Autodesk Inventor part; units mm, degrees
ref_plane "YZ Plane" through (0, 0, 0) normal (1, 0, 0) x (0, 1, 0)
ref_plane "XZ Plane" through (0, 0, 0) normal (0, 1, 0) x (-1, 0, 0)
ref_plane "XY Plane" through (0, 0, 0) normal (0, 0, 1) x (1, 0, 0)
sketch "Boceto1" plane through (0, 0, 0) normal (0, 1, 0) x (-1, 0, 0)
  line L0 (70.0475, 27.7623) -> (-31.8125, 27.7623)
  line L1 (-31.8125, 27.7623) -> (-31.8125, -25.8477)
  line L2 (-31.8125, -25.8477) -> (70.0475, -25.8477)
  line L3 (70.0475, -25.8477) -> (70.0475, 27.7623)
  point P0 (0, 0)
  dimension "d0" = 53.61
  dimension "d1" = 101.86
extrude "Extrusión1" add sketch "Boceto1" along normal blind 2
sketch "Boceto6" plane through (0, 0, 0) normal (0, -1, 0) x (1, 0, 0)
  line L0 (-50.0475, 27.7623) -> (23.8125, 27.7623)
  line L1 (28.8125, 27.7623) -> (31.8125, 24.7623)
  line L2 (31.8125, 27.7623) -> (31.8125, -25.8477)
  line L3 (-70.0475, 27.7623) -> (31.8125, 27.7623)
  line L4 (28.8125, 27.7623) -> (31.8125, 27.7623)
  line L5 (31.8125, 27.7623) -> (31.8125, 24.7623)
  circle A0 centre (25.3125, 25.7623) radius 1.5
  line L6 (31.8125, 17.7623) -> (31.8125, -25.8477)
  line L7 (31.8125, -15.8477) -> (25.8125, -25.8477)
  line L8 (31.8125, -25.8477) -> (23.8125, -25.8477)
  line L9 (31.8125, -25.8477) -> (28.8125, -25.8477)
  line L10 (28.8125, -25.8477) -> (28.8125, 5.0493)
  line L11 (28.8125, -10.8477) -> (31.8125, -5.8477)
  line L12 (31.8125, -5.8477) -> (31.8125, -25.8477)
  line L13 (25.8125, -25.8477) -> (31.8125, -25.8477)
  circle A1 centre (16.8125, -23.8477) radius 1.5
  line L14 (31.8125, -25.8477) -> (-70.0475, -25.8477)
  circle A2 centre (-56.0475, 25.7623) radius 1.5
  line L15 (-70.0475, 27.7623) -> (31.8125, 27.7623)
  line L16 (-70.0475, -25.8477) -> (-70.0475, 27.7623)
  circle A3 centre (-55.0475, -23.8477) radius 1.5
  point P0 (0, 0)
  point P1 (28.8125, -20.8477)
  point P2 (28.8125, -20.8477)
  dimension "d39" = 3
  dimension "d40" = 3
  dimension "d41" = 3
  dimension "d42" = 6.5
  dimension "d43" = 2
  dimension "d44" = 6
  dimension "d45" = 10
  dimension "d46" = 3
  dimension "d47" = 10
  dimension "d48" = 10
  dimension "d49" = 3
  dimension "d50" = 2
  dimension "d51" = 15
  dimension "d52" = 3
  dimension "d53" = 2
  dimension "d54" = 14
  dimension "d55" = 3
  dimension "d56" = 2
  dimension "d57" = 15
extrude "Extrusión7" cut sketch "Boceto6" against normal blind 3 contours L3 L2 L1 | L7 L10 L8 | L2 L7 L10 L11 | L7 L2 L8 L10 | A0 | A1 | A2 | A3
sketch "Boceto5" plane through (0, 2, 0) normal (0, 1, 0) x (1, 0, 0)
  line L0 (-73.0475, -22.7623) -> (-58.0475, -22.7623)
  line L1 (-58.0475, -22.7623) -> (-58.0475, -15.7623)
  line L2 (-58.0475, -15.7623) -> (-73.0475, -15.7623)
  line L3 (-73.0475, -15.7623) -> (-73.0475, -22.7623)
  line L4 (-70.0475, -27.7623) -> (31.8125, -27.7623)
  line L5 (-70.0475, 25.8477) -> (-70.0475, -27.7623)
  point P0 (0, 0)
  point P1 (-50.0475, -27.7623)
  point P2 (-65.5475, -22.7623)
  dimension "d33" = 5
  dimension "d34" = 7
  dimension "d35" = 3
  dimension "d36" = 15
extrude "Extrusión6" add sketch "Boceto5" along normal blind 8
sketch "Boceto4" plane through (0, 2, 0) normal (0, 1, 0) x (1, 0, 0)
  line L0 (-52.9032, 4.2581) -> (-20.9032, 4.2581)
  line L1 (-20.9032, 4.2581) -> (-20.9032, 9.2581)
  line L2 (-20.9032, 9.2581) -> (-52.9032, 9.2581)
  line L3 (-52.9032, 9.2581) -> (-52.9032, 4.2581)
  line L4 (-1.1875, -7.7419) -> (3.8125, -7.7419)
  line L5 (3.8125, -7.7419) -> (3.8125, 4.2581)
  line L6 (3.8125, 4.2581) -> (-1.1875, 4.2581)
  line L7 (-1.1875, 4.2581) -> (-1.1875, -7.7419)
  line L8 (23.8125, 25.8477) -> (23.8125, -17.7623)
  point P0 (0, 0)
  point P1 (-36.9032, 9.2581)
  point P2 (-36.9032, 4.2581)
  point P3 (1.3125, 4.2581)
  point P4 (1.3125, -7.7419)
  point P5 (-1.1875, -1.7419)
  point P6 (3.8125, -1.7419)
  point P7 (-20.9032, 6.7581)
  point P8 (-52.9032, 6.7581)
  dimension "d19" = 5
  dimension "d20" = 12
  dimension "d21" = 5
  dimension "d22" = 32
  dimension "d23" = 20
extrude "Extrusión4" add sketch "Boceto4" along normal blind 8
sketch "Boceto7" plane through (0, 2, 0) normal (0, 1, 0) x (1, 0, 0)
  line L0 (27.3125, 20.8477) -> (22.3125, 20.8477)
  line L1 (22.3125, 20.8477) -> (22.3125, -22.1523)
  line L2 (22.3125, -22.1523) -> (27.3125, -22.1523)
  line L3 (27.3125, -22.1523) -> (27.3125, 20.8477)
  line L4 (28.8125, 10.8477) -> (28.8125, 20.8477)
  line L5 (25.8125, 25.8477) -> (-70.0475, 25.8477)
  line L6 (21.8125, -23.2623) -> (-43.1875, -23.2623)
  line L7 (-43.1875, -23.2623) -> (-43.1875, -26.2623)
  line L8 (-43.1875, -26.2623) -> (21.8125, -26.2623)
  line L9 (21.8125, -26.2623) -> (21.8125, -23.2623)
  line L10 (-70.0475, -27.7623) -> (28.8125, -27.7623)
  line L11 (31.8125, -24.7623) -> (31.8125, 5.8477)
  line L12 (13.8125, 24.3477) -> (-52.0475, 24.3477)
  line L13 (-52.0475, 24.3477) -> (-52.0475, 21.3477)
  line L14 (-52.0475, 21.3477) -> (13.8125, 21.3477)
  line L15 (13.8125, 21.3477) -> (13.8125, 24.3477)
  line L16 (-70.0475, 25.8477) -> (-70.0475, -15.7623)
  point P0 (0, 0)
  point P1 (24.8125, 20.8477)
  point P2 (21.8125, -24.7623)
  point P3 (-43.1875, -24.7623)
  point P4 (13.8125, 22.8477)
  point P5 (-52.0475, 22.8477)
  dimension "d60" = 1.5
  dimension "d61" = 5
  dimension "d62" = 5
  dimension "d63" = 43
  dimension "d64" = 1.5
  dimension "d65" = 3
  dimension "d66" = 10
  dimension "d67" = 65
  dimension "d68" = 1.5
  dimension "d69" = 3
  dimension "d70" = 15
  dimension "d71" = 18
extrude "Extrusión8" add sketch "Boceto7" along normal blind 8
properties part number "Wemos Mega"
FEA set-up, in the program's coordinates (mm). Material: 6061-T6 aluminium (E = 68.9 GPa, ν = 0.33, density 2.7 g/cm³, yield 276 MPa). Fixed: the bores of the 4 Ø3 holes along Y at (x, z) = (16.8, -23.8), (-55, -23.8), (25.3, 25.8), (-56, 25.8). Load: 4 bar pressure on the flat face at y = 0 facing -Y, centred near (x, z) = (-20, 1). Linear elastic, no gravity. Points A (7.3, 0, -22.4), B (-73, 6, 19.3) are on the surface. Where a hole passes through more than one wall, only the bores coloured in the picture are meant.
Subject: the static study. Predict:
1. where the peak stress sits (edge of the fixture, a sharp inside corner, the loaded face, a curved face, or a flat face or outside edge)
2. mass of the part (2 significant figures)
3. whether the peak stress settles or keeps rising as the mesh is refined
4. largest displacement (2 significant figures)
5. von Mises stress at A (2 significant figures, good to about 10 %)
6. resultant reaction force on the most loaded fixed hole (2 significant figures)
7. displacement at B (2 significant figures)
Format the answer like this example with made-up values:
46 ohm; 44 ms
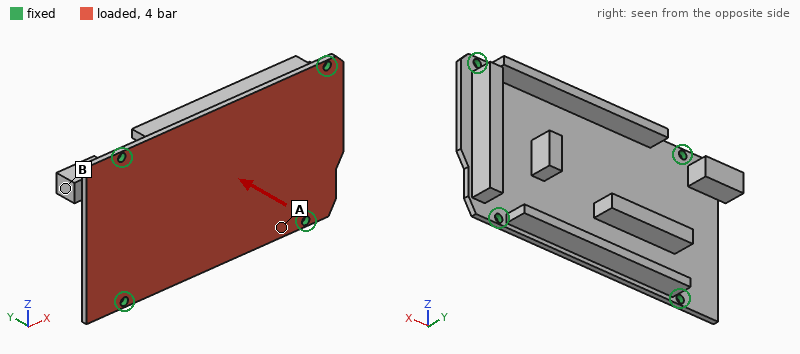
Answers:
edge of the fixture; 49 g; keeps rising; 0.34 mm; 43 MPa; 670 N; 0.093 mm
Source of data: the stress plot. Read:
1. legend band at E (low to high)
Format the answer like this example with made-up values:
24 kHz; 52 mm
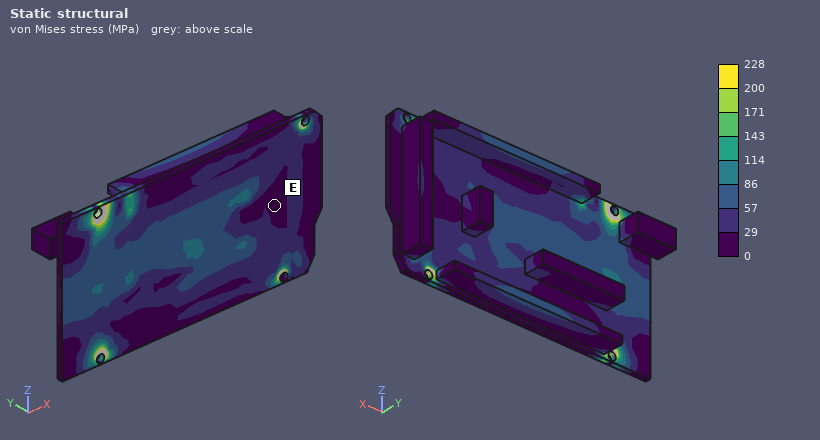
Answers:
0 to 29 MPa
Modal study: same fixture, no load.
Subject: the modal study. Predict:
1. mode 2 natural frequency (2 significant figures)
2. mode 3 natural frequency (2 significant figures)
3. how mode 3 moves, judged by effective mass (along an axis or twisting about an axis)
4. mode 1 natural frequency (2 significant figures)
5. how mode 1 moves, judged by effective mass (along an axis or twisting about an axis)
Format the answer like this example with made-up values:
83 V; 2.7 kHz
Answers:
3100 Hz; 4100 Hz; twisting about X; 2400 Hz; along Y
